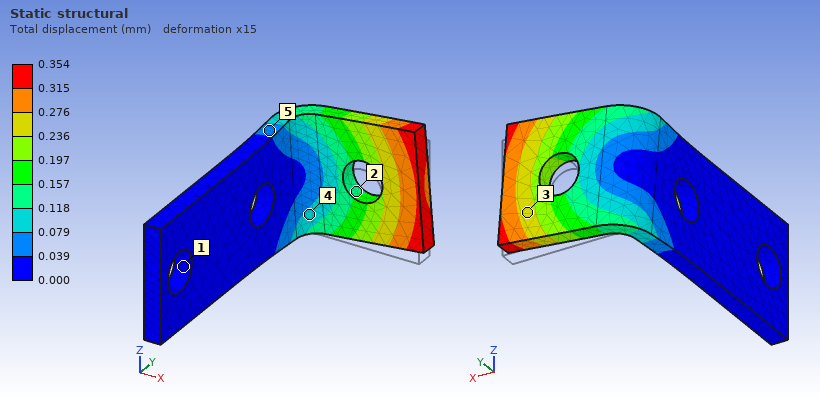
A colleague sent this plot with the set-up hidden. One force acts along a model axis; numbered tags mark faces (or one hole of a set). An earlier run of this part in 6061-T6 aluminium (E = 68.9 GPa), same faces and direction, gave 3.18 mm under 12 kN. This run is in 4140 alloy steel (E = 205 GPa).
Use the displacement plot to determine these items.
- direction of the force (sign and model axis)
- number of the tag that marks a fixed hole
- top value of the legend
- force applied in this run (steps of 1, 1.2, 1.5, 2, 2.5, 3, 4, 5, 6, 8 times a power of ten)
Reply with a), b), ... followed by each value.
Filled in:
a) +Z
b) 1
c) 0.354 mm
d) 4 kN
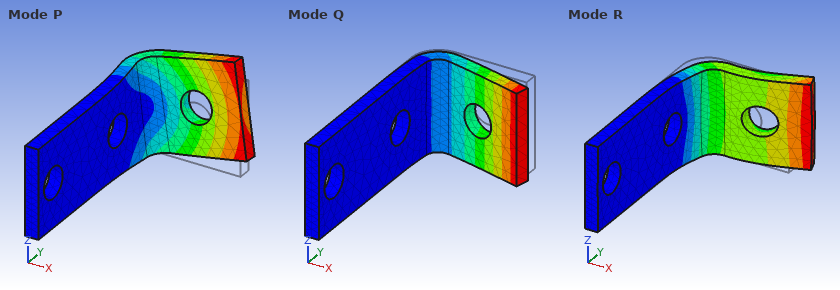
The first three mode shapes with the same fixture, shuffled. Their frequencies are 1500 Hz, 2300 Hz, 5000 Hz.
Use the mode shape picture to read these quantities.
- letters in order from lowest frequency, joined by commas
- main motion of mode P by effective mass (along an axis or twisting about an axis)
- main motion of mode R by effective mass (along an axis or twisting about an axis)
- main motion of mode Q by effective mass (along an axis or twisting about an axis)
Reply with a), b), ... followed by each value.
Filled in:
a) Q, P, R
b) along Z
c) along X
d) along Y
